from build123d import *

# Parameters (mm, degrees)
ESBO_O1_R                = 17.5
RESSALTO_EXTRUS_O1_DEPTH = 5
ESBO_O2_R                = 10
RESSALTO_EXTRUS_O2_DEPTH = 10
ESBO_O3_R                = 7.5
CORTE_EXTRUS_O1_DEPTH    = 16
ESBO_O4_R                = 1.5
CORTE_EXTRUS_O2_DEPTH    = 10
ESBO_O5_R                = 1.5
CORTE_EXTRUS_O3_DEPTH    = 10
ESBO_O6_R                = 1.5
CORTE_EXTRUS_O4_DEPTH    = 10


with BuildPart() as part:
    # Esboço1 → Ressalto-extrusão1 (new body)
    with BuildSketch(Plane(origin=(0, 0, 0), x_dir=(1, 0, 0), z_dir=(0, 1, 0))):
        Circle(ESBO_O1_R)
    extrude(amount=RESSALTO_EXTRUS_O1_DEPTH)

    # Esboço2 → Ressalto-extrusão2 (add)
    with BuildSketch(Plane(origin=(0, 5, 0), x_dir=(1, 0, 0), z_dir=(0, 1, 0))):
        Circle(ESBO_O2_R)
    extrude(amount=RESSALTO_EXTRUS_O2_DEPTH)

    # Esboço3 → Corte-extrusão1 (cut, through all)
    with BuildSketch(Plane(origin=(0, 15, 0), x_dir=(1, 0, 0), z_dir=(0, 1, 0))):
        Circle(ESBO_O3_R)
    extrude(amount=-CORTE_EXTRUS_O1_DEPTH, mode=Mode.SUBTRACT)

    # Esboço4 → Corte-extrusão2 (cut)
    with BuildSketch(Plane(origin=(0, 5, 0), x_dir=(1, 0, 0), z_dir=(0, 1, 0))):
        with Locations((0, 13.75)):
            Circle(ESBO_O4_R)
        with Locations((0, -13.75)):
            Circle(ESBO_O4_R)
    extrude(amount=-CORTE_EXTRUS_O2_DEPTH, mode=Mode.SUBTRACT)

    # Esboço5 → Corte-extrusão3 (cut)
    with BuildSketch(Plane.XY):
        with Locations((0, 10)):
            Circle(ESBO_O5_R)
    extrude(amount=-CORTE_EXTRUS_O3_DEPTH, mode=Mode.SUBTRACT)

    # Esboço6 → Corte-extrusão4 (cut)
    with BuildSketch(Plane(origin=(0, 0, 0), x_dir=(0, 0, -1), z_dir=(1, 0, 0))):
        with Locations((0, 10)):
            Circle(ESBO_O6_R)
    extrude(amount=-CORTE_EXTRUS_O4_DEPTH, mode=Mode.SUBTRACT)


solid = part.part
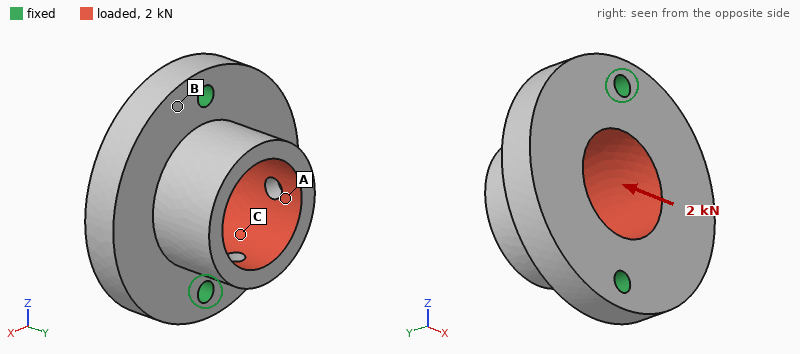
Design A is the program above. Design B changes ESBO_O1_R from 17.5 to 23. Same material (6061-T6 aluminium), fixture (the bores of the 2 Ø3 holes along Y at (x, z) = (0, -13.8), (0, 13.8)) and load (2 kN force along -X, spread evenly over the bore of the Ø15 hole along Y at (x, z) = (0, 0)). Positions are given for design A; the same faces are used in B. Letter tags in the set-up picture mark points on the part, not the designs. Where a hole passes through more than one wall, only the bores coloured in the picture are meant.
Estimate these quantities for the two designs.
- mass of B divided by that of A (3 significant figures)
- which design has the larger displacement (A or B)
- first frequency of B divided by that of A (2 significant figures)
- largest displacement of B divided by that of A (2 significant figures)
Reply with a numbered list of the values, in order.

1. 1.67
2. A
3. 0.71
4. 0.91
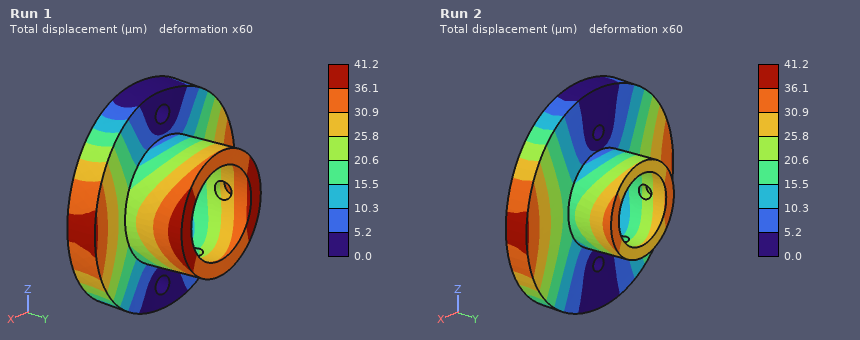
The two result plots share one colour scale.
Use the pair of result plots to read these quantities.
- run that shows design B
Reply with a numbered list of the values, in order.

1. Run 2
